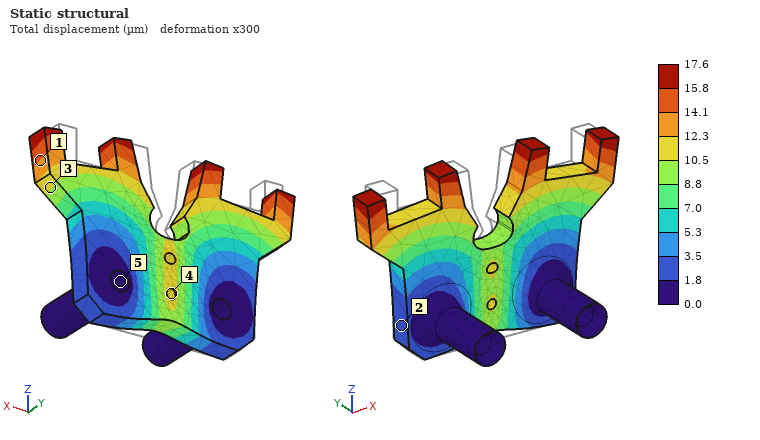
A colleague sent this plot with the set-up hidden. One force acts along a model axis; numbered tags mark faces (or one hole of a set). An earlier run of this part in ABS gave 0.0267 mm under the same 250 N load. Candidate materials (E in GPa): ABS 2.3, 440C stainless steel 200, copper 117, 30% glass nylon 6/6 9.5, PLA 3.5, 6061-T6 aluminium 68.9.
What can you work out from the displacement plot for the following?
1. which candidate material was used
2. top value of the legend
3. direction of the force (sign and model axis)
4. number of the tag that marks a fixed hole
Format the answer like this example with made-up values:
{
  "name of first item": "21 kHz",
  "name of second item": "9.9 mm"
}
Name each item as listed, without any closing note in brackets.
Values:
{
  "which candidate material was used": "PLA",
  "top value of the legend": "17.6 µm",
  "direction of the force": "+Z",
  "number of the tag that marks a fixed hole": "5"
}
